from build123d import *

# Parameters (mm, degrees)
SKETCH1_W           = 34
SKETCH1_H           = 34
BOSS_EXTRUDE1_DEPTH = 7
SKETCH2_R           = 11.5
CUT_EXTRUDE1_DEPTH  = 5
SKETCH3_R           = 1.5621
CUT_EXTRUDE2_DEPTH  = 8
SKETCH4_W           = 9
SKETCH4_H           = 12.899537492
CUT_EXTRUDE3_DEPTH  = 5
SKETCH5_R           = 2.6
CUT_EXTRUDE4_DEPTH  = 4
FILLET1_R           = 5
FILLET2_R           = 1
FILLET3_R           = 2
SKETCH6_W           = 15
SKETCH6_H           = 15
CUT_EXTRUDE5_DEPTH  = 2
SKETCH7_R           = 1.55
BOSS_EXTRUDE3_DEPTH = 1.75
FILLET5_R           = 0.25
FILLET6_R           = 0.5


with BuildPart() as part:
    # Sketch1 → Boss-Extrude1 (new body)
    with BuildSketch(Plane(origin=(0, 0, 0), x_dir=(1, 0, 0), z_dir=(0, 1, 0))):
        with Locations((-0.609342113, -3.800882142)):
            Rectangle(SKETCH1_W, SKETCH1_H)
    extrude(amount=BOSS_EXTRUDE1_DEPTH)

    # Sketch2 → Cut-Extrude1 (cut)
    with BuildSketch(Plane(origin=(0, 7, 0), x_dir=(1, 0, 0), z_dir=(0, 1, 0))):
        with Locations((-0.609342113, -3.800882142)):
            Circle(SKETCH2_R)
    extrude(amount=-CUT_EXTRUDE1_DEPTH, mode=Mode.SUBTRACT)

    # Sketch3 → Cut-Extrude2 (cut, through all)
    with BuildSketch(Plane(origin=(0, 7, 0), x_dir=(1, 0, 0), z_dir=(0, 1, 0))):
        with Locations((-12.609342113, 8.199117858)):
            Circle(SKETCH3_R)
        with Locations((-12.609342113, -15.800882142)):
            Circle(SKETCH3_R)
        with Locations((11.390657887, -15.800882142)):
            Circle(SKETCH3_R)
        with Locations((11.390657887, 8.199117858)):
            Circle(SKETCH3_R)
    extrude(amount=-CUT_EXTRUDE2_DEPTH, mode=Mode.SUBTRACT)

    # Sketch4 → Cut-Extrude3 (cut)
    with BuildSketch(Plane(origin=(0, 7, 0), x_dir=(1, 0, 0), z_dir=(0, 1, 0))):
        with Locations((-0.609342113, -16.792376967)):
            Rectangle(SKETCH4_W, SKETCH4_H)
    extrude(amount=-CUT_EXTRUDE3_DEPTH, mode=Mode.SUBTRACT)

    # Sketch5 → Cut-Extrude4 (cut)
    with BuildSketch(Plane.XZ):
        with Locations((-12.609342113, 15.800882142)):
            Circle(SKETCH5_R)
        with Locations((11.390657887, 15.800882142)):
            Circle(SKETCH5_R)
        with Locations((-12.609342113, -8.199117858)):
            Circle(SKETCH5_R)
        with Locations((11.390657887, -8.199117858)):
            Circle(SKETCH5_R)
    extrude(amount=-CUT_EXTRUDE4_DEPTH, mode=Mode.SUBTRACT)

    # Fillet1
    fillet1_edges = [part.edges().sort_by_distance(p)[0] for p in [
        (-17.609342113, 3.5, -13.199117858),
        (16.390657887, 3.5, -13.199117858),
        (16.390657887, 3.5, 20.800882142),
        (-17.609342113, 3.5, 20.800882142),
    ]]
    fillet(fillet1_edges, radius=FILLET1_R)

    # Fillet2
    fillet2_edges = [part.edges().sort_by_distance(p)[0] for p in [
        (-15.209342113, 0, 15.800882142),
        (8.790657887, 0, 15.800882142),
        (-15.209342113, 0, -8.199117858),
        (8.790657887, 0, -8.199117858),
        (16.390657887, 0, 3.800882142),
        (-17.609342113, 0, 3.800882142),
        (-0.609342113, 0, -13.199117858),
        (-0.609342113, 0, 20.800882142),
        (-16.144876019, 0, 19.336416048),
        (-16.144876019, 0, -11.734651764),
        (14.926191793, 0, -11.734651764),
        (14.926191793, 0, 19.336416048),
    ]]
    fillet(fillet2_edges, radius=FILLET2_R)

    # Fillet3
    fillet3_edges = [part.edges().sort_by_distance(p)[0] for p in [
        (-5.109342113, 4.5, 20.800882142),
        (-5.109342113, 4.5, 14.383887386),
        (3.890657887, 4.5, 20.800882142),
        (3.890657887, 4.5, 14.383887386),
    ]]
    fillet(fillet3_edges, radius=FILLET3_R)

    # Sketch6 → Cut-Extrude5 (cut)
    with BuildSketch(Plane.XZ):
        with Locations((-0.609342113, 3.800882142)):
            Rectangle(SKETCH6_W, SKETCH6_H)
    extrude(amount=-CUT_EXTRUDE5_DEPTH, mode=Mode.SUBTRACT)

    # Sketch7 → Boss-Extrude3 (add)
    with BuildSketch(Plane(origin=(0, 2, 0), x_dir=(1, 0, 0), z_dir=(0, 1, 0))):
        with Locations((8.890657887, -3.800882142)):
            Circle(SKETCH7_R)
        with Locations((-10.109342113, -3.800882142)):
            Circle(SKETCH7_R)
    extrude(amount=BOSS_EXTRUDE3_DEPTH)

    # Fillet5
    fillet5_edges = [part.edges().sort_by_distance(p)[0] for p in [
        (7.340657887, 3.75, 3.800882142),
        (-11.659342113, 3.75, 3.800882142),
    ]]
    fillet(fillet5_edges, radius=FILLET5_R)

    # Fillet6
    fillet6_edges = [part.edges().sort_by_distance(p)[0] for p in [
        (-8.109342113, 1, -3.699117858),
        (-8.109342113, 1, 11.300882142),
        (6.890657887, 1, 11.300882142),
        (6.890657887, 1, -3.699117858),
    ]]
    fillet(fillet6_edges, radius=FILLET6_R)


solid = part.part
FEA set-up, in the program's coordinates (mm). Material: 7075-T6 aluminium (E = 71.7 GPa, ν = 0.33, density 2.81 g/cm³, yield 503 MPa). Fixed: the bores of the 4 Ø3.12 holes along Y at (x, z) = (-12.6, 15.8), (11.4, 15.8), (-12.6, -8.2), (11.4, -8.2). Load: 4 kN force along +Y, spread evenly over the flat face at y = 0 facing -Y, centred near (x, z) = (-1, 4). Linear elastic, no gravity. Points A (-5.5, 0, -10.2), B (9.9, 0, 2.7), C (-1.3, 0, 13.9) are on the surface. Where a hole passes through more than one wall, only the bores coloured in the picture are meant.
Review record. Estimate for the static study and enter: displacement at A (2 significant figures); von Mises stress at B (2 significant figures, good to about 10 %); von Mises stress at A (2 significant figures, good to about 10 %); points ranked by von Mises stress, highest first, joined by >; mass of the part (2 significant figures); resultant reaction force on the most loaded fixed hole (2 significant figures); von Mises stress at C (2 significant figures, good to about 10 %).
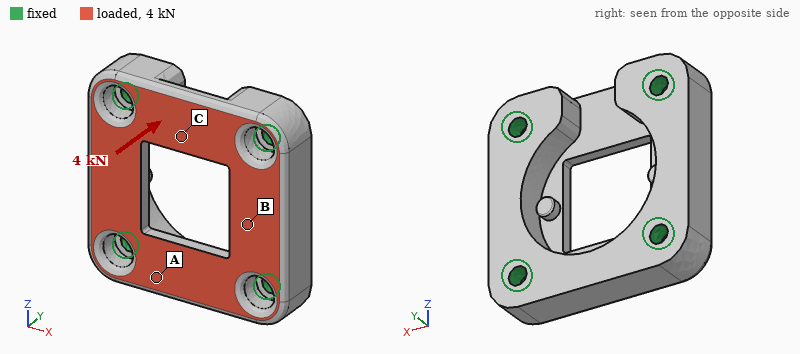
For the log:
6.6 µm
48 MPa
22 MPa
C > B > A
13 g
1.2 kN
79 MPa
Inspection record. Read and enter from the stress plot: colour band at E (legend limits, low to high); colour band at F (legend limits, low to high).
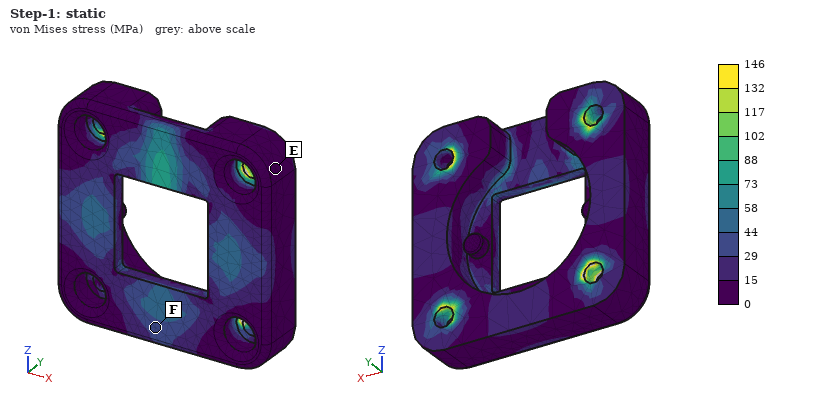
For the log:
0 to 15 MPa
29 to 44 MPa
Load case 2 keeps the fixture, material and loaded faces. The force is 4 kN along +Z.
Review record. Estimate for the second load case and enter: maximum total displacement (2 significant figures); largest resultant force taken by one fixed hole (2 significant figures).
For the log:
20 µm
1.1 kN
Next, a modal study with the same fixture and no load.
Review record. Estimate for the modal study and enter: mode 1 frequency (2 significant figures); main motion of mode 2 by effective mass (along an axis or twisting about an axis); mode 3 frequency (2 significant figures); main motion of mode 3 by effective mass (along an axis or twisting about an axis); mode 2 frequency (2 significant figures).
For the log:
31 kHz
along X
36 kHz
along Y
34 kHz
